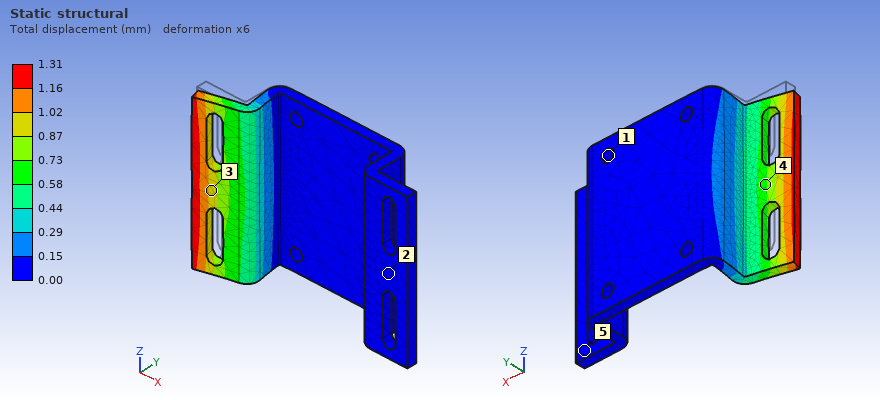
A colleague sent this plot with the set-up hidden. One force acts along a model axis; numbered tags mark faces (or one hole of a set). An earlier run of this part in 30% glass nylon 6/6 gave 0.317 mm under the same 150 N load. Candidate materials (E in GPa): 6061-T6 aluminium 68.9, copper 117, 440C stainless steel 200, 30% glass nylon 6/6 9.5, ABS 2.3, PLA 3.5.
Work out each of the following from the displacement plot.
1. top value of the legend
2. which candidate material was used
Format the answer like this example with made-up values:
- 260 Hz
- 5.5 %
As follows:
- 1.31 mm
- ABS
